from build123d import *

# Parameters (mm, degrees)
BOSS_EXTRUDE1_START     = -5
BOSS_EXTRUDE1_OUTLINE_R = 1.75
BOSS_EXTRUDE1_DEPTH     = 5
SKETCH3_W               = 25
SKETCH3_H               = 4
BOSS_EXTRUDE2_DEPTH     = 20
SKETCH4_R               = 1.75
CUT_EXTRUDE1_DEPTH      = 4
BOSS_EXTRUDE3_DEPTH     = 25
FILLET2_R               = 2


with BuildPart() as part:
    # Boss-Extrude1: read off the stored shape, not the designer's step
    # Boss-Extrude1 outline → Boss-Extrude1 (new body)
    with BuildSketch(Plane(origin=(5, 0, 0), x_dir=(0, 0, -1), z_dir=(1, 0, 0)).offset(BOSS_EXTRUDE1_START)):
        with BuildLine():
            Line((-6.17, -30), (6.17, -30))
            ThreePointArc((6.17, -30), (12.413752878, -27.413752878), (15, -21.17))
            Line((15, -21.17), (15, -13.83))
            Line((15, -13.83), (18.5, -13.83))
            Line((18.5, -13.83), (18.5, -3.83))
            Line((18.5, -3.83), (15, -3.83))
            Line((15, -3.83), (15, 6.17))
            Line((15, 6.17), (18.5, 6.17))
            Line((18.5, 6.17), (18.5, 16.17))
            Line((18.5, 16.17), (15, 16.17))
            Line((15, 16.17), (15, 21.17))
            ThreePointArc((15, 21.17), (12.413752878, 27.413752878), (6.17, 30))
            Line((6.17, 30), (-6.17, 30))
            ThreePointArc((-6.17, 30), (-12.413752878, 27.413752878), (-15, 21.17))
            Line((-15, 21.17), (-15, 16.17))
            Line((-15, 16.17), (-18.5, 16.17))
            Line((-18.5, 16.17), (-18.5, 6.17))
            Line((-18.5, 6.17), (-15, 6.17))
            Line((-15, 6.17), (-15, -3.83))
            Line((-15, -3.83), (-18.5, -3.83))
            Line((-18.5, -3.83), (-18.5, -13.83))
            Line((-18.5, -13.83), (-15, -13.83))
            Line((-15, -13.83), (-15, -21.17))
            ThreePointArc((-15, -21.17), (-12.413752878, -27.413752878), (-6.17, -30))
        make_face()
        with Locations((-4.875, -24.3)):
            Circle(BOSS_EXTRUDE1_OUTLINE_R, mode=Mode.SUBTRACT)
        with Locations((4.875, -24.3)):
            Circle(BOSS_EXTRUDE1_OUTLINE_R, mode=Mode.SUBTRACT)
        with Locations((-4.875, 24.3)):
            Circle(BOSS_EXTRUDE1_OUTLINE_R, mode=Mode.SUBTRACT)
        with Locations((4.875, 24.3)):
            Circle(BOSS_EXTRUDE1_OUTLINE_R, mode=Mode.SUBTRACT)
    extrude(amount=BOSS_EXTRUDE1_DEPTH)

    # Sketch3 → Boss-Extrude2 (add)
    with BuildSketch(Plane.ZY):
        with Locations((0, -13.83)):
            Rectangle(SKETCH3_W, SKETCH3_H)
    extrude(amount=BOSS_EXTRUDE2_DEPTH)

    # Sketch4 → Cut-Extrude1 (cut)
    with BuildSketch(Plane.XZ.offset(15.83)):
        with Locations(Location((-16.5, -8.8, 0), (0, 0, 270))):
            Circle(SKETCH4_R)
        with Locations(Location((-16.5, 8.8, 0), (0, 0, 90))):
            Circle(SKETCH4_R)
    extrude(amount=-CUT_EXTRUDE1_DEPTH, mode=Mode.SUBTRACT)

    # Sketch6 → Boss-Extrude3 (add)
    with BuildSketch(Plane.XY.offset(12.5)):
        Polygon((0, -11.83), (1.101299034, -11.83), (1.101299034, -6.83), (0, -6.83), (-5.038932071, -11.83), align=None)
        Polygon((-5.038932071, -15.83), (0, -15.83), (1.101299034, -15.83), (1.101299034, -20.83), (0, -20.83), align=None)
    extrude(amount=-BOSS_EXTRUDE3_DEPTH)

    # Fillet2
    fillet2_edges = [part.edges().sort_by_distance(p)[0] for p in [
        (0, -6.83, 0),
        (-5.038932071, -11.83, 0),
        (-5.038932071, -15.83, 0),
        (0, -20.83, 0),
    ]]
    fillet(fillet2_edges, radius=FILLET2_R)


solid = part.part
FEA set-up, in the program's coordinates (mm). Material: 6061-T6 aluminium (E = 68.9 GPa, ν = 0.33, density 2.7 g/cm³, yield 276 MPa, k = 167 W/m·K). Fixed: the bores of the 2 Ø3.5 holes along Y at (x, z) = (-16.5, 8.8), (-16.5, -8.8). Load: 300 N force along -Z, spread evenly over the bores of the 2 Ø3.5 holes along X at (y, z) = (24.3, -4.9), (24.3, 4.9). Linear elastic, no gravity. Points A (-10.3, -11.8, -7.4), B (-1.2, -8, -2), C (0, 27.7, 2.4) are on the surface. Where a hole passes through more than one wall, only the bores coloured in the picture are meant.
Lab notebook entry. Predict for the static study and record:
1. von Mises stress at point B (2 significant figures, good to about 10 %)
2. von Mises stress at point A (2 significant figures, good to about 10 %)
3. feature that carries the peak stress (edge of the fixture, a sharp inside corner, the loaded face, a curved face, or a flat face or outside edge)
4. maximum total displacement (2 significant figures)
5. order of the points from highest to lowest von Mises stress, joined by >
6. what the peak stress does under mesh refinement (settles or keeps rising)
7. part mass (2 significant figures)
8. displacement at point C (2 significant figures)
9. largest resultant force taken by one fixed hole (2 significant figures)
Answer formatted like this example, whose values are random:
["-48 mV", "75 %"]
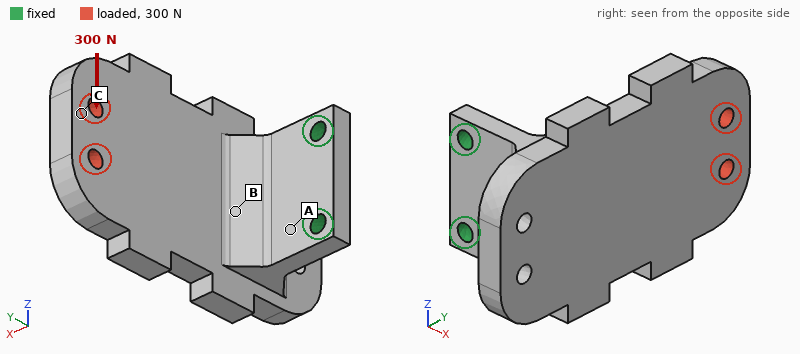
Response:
["32 MPa", "65 MPa", "edge of the fixture", "0.19 mm", "A > B > C", "keeps rising", "32 g", "0.18 mm", "690 N"]
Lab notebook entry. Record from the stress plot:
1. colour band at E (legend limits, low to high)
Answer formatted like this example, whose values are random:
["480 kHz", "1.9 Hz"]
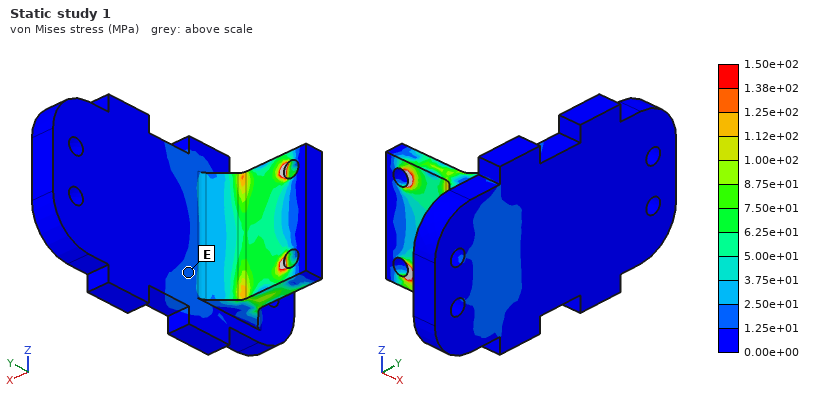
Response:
["1.25e+01 to 2.50e+01 MPa"]
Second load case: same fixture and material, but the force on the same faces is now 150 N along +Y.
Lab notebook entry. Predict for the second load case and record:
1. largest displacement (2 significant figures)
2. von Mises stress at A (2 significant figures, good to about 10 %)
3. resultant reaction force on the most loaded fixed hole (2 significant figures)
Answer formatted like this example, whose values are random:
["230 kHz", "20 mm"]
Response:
["0.12 mm", "28 MPa", "75 N"]
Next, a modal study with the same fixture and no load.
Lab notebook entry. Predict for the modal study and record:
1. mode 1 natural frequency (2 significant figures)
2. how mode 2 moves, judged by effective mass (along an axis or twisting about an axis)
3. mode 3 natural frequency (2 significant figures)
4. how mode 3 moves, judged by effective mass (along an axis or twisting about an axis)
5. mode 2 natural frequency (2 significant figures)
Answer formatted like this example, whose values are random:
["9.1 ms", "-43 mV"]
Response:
["1000 Hz", "along Z", "4200 Hz", "along Y", "2300 Hz"]
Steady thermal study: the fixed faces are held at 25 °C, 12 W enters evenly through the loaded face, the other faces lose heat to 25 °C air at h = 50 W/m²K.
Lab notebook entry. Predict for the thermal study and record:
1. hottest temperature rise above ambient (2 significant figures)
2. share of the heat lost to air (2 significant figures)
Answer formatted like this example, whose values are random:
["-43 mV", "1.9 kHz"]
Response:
["24 K", "27 %"]
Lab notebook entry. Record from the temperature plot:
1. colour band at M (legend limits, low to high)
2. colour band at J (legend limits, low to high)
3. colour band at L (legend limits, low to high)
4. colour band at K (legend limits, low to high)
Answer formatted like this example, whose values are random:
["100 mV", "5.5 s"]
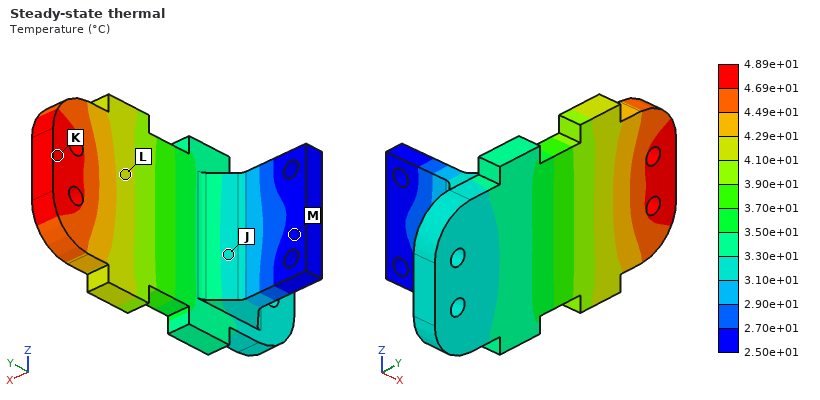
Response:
["2.50e+01 to 2.70e+01 °C", "3.10e+01 to 3.30e+01 °C", "4.10e+01 to 4.29e+01 °C", "4.69e+01 to 4.89e+01 °C"]
